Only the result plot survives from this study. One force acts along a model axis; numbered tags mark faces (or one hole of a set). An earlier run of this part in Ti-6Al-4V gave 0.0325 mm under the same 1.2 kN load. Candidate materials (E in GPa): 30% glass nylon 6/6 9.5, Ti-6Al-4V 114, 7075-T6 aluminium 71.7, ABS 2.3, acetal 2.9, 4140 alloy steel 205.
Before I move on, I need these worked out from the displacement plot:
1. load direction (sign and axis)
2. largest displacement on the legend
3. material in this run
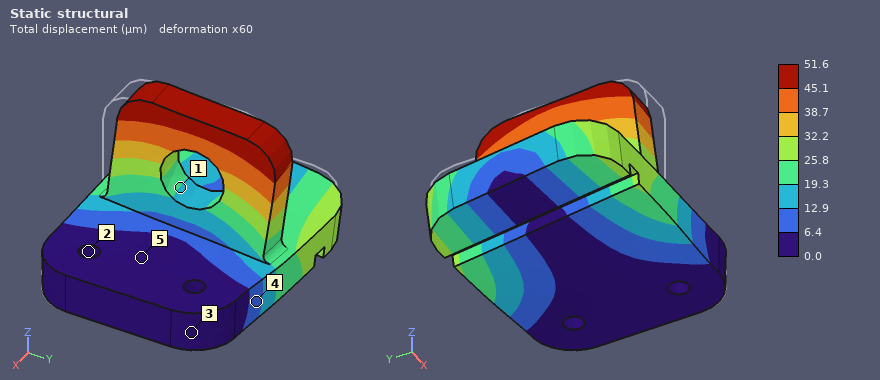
+Y
51.6 µm
7075-T6 aluminium
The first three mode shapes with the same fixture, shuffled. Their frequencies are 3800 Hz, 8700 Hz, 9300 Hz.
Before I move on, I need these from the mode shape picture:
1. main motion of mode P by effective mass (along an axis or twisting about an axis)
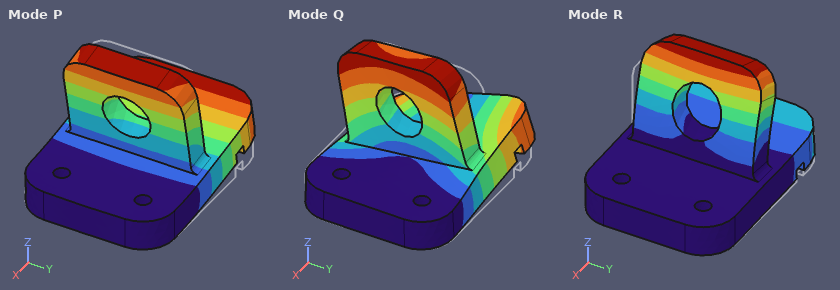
along Z
